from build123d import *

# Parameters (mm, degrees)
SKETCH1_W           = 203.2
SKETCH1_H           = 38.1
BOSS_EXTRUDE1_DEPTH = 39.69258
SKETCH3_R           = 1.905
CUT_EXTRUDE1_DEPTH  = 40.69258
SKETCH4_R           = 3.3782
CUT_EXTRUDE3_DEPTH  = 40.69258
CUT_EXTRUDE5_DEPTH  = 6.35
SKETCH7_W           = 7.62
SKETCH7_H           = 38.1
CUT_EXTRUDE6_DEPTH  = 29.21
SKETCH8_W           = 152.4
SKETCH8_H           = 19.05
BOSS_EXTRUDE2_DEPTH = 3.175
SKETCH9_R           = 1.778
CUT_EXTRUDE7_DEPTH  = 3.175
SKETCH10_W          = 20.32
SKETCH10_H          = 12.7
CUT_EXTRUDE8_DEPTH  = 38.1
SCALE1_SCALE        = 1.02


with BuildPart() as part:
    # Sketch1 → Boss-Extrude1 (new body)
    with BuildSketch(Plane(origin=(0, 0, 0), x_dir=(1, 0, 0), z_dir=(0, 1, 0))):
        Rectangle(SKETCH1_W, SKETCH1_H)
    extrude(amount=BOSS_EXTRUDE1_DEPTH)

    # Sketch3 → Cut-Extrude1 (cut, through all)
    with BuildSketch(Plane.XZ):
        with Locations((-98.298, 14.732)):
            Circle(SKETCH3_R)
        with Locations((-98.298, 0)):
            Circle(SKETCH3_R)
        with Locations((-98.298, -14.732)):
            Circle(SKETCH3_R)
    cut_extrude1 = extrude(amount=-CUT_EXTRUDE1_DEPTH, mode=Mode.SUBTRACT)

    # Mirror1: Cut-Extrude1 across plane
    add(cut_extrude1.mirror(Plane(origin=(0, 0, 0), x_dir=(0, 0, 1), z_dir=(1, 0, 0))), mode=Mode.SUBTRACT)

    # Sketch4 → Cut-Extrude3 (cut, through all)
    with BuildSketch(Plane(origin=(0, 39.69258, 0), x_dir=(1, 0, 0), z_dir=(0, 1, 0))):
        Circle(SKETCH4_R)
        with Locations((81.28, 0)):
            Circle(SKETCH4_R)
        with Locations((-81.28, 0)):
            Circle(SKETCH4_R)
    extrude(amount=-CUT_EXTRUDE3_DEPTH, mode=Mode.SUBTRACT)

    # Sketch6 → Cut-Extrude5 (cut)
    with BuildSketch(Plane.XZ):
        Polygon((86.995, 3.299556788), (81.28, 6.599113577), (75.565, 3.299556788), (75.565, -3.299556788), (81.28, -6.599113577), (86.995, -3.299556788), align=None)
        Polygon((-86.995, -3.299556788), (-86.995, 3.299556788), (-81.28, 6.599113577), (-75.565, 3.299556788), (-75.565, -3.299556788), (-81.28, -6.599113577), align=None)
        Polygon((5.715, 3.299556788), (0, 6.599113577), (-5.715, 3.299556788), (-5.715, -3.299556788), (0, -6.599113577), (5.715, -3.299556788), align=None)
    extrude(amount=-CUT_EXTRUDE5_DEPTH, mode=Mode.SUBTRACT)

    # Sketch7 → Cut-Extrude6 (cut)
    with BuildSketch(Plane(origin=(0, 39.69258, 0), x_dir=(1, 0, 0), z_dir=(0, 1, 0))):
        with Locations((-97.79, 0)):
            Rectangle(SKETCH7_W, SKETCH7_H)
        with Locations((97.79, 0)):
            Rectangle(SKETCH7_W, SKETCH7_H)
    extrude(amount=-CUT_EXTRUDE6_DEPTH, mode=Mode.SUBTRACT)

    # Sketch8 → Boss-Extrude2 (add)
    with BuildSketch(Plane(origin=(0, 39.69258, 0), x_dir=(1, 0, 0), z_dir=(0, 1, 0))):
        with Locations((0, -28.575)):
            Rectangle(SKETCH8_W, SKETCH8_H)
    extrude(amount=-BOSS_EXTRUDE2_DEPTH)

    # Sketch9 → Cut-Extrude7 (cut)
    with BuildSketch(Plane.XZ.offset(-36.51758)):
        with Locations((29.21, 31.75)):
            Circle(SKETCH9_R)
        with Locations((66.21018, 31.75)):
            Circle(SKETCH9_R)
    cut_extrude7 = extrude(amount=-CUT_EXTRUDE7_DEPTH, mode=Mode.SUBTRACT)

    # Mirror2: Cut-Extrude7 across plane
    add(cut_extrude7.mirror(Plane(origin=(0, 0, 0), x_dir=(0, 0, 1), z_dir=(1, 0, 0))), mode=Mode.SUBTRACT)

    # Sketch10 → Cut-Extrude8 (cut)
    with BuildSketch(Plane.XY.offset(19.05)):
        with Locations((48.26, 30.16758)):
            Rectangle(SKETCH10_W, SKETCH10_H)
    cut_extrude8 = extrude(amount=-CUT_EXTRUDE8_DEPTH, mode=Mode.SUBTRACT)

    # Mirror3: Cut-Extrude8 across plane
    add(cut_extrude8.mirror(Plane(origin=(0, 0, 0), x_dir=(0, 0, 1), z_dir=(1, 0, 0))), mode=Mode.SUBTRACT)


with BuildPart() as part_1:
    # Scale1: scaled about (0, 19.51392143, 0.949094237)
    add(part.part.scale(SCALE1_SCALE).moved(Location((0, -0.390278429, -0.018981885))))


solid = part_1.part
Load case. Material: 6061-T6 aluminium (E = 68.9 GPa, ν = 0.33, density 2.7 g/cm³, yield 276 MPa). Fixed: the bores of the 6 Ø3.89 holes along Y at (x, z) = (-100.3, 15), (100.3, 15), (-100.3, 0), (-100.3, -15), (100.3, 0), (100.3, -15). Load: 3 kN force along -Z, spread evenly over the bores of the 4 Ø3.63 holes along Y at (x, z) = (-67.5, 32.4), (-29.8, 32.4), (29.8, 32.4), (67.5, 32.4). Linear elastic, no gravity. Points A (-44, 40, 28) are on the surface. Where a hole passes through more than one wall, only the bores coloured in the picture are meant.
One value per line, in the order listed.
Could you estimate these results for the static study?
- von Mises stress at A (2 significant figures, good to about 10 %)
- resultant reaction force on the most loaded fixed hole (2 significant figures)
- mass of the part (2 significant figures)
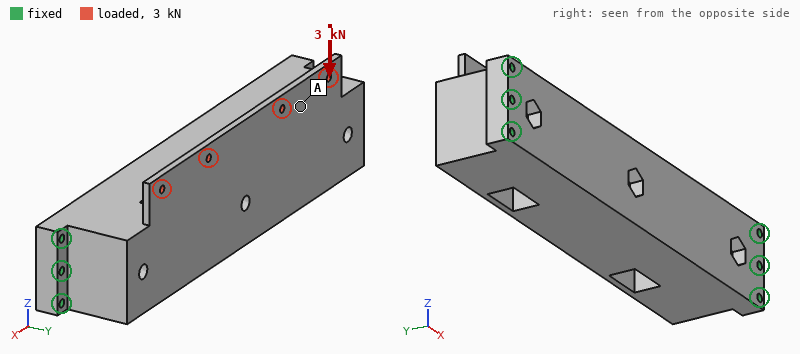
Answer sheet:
5.7 MPa
2.1 kN
780 g
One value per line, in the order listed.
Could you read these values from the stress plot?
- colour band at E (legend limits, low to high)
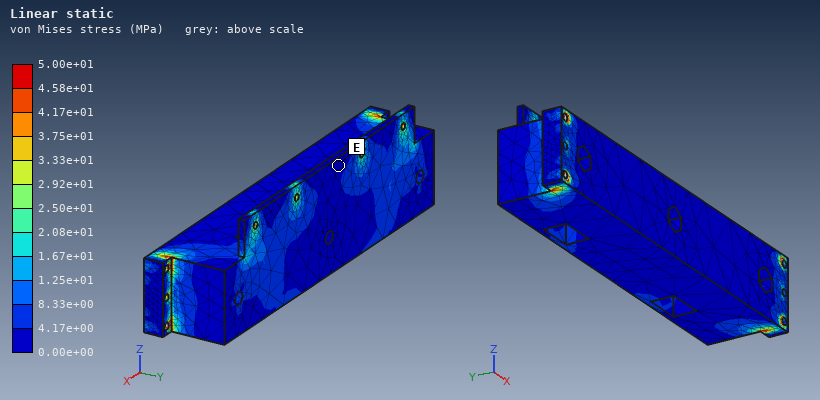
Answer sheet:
0.00e+00 to 4.17e+00 MPa
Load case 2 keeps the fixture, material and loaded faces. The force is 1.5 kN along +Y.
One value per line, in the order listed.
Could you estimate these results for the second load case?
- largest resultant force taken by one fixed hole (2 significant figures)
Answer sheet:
1.1 kN
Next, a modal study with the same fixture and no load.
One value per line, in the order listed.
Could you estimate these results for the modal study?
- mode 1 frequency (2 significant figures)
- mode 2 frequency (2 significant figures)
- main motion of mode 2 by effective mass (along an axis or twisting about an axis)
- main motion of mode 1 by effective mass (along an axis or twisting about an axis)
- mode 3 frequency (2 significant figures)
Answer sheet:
2600 Hz
2900 Hz
along Z
along Y
4100 Hz
